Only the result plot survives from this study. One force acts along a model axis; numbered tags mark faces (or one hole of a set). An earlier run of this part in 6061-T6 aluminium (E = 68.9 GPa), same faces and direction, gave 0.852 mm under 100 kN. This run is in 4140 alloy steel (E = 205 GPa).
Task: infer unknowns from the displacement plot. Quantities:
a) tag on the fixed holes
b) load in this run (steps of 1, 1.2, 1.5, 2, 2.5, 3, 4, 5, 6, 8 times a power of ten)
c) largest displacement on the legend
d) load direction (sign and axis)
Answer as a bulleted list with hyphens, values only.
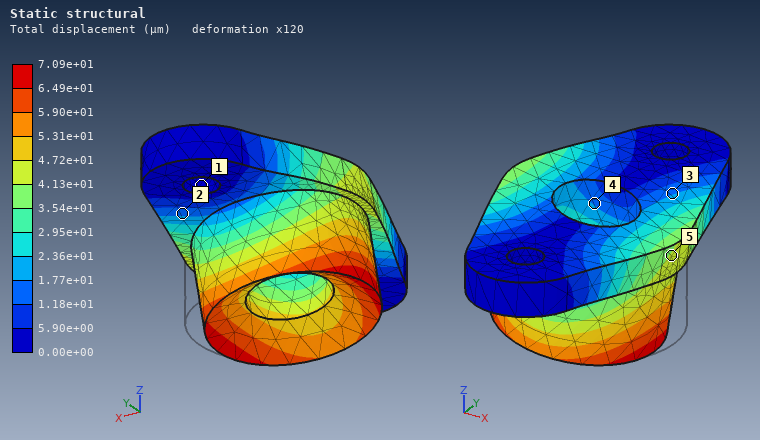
- 1
- 25 kN
- 7.09e+01 µm
- -X
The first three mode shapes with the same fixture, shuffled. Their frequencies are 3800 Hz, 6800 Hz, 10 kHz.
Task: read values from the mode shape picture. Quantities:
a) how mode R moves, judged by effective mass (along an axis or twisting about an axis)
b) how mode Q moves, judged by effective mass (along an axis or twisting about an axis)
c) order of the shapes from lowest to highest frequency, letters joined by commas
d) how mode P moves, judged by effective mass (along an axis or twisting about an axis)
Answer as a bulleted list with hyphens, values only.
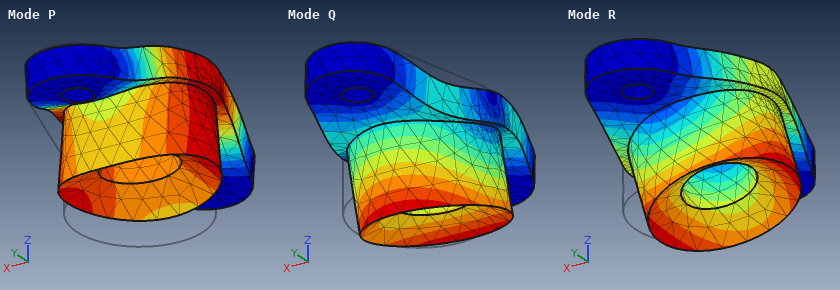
- along X
- along Y
- R, P, Q
- along Z
